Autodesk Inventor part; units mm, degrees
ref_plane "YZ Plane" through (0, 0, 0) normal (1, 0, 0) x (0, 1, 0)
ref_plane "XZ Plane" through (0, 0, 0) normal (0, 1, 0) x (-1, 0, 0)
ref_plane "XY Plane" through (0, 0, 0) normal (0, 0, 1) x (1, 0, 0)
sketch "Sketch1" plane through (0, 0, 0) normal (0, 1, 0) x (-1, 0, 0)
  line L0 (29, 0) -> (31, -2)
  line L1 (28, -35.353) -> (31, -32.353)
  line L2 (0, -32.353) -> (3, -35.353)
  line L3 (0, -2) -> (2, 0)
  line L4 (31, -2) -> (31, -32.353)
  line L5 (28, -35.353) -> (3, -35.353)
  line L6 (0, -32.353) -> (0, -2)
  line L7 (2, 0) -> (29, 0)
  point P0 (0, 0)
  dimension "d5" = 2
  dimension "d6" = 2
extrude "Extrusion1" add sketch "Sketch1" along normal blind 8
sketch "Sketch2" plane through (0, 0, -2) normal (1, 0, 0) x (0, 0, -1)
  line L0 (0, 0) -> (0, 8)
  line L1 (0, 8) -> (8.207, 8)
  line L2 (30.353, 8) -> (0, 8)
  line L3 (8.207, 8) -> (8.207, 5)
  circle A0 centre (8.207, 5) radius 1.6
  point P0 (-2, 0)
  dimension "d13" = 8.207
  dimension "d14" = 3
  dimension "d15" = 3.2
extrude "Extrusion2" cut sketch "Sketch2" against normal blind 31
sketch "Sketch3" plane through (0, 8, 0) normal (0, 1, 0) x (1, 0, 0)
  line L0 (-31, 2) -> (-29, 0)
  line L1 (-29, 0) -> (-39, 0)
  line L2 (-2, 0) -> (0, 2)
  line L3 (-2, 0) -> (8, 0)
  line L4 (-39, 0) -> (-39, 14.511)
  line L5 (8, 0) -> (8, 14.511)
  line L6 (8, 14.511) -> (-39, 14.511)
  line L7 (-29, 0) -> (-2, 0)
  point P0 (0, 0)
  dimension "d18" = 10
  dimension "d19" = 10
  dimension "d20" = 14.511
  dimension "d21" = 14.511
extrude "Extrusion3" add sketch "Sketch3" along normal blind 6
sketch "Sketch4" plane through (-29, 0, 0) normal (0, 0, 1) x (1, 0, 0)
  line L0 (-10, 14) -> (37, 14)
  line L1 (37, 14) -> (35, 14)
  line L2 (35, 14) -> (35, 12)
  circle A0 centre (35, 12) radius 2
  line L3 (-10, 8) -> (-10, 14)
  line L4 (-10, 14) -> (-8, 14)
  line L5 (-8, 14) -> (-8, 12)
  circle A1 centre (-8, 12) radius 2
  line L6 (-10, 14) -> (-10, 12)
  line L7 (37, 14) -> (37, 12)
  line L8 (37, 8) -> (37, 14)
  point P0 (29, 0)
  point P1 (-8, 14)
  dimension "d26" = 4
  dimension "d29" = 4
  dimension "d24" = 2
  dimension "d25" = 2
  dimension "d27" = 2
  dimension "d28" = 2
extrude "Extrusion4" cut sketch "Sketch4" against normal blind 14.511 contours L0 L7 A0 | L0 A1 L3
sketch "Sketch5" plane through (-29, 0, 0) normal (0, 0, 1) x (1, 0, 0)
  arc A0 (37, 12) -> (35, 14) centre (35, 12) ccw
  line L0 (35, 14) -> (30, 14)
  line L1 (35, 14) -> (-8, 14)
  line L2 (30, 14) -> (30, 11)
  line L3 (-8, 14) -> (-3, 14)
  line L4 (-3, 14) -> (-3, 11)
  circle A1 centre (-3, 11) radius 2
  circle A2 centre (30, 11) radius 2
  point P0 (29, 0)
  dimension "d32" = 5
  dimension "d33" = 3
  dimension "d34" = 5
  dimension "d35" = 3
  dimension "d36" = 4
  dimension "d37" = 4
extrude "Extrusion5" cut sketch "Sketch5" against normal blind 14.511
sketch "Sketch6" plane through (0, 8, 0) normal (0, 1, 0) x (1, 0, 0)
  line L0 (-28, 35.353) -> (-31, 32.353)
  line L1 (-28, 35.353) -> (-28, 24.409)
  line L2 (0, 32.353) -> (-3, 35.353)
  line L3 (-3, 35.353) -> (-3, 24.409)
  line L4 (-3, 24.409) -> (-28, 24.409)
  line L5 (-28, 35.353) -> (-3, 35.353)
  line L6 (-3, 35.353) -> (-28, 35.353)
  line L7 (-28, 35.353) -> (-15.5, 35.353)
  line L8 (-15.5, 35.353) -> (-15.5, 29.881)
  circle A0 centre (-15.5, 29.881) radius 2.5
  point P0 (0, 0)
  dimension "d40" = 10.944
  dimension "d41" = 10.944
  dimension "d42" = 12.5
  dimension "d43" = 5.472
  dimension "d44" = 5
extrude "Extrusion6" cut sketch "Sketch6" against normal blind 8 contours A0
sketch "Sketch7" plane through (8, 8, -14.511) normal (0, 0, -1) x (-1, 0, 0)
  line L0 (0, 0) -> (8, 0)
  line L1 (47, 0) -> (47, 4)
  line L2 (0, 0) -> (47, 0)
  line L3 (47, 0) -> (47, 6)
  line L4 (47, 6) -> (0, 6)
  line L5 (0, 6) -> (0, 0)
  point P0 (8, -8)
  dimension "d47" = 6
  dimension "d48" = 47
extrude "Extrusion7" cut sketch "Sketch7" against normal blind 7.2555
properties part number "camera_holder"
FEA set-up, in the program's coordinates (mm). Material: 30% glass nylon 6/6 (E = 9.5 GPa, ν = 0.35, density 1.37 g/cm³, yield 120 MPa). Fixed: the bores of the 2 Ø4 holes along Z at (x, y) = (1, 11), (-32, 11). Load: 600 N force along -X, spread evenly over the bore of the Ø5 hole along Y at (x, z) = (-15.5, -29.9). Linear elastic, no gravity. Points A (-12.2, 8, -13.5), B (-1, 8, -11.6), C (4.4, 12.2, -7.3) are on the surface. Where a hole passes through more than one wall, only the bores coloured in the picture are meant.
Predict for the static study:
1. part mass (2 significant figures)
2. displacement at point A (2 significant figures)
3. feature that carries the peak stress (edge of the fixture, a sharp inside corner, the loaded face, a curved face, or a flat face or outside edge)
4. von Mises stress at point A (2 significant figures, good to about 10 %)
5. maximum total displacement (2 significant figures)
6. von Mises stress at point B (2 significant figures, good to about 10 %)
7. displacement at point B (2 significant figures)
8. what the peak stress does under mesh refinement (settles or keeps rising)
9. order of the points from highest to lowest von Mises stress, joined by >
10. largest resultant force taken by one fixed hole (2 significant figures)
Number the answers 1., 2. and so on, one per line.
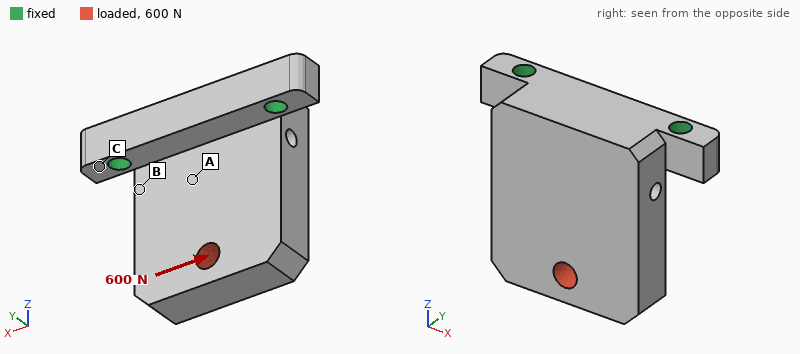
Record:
1. 14 g
2. 0.043 mm
3. a sharp inside corner
4. 12 MPa
5. 0.14 mm
6. 23 MPa
7. 0.052 mm
8. keeps rising
9. B > A > C
10. 640 N
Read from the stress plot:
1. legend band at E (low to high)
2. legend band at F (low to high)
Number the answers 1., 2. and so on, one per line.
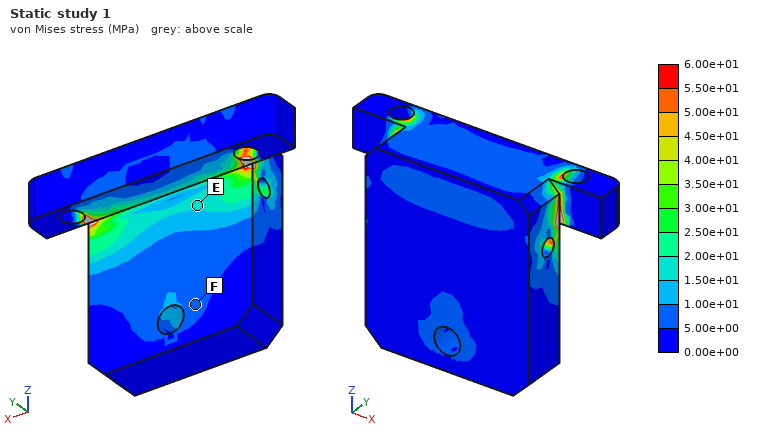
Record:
1. 1.50e+01 to 2.00e+01 MPa
2. 5.00e+00 to 1.00e+01 MPa
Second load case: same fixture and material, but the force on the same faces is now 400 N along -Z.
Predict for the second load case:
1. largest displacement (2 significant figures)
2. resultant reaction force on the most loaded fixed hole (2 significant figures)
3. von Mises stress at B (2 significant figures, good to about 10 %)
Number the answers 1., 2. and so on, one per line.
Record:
1. 0.12 mm
2. 200 N
3. 5.6 MPa
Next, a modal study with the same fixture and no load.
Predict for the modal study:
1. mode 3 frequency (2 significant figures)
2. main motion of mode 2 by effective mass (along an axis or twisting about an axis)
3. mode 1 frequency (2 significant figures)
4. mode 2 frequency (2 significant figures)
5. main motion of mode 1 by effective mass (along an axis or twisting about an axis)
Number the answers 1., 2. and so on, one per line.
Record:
1. 6800 Hz
2. along X
3. 1800 Hz
4. 4900 Hz
5. along Y
